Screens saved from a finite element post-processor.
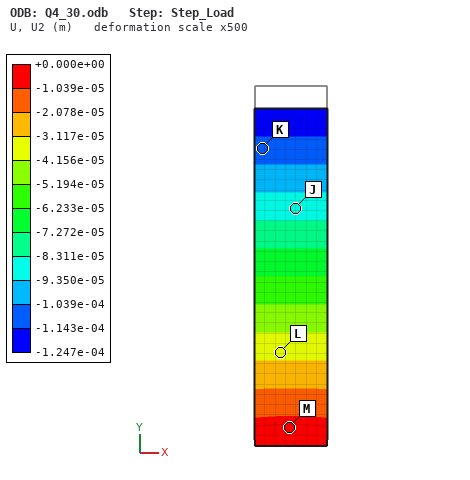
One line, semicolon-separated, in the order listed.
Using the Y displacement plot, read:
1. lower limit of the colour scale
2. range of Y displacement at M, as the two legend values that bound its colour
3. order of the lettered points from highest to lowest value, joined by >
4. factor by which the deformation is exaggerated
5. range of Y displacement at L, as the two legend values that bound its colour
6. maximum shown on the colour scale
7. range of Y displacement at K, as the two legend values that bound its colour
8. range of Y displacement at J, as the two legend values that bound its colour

-1.247e-04 m; -1.039e-05 to +0.000e+00 m; M > L > J > K; 500; -4.156e-05 to -3.117e-05 m; +0.000e+00 m; -1.143e-04 to -1.039e-04 m; -9.350e-05 to -8.311e-05 m
